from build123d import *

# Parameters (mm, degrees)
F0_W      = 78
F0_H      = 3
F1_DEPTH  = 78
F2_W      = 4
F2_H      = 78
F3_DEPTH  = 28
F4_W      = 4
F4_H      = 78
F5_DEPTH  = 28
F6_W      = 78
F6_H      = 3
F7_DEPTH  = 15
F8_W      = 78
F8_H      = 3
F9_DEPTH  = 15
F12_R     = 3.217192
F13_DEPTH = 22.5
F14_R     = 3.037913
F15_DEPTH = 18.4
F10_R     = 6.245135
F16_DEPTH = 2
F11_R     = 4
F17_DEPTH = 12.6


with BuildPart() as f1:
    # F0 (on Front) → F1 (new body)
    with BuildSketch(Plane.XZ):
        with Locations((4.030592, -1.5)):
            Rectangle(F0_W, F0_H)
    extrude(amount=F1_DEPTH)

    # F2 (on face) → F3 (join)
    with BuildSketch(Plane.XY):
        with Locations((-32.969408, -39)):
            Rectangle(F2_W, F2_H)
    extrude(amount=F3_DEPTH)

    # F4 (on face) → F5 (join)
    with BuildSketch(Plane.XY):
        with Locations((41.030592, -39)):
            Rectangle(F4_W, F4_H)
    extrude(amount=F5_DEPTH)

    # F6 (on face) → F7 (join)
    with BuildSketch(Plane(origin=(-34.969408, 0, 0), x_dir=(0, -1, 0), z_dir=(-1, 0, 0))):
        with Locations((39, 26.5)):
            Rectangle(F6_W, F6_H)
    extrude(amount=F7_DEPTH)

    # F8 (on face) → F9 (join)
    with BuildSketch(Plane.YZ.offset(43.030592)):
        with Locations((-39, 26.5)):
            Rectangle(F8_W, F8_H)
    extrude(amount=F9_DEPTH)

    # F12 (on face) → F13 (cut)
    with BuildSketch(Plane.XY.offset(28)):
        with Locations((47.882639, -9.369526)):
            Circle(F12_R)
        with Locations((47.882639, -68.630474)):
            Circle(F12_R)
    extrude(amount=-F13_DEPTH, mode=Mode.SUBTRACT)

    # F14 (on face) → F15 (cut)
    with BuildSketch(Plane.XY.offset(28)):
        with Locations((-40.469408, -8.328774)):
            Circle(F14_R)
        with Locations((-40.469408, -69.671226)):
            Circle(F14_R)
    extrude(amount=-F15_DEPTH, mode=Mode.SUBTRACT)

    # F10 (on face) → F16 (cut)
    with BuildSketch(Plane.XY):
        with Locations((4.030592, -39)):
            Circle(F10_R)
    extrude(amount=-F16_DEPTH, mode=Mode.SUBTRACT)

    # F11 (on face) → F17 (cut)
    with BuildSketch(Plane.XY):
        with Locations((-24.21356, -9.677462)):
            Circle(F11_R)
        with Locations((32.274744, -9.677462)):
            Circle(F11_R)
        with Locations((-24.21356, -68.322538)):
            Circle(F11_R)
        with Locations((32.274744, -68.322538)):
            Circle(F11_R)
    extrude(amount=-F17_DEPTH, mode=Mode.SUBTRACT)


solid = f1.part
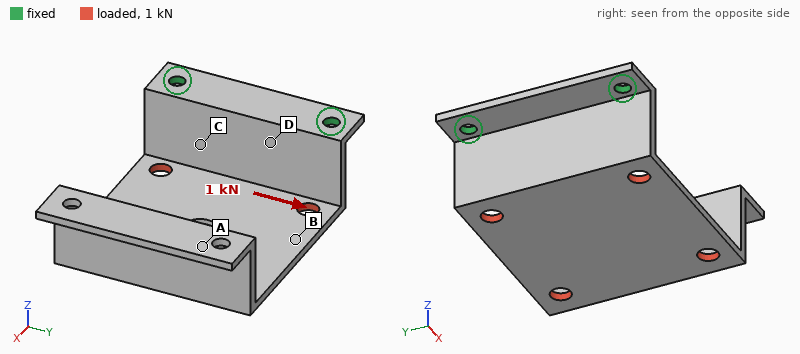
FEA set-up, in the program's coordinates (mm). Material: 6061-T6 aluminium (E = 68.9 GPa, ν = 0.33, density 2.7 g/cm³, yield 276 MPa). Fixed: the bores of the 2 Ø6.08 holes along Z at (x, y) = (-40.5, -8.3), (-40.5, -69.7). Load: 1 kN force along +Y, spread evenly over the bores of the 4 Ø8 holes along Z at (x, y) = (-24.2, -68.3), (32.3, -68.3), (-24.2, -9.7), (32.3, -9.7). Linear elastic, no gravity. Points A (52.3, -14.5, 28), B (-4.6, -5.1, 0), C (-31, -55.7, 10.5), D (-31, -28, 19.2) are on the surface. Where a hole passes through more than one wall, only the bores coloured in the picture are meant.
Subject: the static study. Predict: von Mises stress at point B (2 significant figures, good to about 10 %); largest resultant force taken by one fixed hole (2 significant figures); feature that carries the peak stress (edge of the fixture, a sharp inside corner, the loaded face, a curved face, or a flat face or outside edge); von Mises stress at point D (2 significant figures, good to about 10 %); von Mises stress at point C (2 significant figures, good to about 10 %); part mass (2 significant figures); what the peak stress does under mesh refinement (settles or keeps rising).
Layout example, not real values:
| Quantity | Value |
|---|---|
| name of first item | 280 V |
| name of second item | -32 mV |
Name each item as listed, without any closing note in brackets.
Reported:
| Quantity | Value |
|---|---|
| von Mises stress at point B | 26 MPa |
| largest resultant force taken by one fixed hole | 970 N |
| feature that carries the peak stress | edge of the fixture |
| von Mises stress at point D | 79 MPa |
| von Mises stress at point C | 91 MPa |
| part mass | 110 g |
| what the peak stress does under mesh refinement | keeps rising |
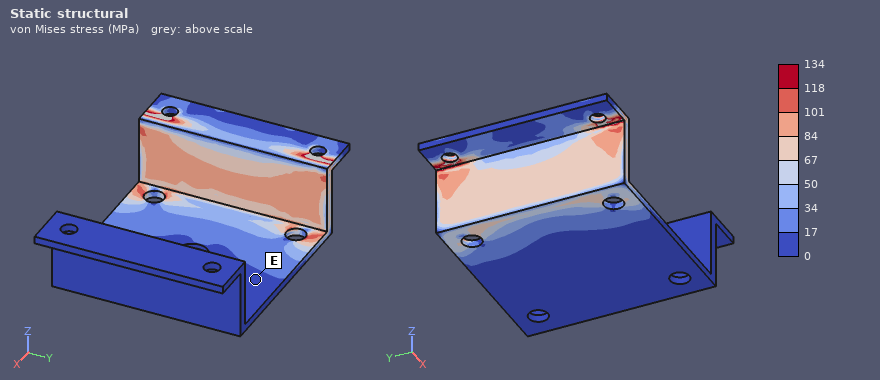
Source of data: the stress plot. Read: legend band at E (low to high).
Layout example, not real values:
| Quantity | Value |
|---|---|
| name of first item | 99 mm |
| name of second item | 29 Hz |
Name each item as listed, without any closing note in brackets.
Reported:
| Quantity | Value |
|---|---|
| legend band at E | 0 to 17 MPa |
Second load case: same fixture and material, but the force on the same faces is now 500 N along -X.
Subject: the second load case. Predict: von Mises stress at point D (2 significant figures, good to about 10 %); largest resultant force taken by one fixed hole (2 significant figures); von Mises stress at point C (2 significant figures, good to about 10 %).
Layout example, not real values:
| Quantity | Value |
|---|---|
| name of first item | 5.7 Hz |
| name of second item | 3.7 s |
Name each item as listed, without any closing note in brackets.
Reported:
| Quantity | Value |
|---|---|
| von Mises stress at point D | 36 MPa |
| largest resultant force taken by one fixed hole | 250 N |
| von Mises stress at point C | 24 MPa |
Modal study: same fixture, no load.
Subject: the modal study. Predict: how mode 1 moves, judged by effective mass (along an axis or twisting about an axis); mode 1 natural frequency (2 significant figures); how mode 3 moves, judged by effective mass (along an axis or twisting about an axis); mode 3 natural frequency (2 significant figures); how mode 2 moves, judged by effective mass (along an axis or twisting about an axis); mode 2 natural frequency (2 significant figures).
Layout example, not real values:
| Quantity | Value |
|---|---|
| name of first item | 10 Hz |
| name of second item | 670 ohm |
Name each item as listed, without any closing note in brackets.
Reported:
| Quantity | Value |
|---|---|
| how mode 1 moves, judged by effective mass | along Z |
| mode 1 natural frequency | 160 Hz |
| how mode 3 moves, judged by effective mass | along X |
| mode 3 natural frequency | 560 Hz |
| how mode 2 moves, judged by effective mass | along Y |
| mode 2 natural frequency | 360 Hz |
